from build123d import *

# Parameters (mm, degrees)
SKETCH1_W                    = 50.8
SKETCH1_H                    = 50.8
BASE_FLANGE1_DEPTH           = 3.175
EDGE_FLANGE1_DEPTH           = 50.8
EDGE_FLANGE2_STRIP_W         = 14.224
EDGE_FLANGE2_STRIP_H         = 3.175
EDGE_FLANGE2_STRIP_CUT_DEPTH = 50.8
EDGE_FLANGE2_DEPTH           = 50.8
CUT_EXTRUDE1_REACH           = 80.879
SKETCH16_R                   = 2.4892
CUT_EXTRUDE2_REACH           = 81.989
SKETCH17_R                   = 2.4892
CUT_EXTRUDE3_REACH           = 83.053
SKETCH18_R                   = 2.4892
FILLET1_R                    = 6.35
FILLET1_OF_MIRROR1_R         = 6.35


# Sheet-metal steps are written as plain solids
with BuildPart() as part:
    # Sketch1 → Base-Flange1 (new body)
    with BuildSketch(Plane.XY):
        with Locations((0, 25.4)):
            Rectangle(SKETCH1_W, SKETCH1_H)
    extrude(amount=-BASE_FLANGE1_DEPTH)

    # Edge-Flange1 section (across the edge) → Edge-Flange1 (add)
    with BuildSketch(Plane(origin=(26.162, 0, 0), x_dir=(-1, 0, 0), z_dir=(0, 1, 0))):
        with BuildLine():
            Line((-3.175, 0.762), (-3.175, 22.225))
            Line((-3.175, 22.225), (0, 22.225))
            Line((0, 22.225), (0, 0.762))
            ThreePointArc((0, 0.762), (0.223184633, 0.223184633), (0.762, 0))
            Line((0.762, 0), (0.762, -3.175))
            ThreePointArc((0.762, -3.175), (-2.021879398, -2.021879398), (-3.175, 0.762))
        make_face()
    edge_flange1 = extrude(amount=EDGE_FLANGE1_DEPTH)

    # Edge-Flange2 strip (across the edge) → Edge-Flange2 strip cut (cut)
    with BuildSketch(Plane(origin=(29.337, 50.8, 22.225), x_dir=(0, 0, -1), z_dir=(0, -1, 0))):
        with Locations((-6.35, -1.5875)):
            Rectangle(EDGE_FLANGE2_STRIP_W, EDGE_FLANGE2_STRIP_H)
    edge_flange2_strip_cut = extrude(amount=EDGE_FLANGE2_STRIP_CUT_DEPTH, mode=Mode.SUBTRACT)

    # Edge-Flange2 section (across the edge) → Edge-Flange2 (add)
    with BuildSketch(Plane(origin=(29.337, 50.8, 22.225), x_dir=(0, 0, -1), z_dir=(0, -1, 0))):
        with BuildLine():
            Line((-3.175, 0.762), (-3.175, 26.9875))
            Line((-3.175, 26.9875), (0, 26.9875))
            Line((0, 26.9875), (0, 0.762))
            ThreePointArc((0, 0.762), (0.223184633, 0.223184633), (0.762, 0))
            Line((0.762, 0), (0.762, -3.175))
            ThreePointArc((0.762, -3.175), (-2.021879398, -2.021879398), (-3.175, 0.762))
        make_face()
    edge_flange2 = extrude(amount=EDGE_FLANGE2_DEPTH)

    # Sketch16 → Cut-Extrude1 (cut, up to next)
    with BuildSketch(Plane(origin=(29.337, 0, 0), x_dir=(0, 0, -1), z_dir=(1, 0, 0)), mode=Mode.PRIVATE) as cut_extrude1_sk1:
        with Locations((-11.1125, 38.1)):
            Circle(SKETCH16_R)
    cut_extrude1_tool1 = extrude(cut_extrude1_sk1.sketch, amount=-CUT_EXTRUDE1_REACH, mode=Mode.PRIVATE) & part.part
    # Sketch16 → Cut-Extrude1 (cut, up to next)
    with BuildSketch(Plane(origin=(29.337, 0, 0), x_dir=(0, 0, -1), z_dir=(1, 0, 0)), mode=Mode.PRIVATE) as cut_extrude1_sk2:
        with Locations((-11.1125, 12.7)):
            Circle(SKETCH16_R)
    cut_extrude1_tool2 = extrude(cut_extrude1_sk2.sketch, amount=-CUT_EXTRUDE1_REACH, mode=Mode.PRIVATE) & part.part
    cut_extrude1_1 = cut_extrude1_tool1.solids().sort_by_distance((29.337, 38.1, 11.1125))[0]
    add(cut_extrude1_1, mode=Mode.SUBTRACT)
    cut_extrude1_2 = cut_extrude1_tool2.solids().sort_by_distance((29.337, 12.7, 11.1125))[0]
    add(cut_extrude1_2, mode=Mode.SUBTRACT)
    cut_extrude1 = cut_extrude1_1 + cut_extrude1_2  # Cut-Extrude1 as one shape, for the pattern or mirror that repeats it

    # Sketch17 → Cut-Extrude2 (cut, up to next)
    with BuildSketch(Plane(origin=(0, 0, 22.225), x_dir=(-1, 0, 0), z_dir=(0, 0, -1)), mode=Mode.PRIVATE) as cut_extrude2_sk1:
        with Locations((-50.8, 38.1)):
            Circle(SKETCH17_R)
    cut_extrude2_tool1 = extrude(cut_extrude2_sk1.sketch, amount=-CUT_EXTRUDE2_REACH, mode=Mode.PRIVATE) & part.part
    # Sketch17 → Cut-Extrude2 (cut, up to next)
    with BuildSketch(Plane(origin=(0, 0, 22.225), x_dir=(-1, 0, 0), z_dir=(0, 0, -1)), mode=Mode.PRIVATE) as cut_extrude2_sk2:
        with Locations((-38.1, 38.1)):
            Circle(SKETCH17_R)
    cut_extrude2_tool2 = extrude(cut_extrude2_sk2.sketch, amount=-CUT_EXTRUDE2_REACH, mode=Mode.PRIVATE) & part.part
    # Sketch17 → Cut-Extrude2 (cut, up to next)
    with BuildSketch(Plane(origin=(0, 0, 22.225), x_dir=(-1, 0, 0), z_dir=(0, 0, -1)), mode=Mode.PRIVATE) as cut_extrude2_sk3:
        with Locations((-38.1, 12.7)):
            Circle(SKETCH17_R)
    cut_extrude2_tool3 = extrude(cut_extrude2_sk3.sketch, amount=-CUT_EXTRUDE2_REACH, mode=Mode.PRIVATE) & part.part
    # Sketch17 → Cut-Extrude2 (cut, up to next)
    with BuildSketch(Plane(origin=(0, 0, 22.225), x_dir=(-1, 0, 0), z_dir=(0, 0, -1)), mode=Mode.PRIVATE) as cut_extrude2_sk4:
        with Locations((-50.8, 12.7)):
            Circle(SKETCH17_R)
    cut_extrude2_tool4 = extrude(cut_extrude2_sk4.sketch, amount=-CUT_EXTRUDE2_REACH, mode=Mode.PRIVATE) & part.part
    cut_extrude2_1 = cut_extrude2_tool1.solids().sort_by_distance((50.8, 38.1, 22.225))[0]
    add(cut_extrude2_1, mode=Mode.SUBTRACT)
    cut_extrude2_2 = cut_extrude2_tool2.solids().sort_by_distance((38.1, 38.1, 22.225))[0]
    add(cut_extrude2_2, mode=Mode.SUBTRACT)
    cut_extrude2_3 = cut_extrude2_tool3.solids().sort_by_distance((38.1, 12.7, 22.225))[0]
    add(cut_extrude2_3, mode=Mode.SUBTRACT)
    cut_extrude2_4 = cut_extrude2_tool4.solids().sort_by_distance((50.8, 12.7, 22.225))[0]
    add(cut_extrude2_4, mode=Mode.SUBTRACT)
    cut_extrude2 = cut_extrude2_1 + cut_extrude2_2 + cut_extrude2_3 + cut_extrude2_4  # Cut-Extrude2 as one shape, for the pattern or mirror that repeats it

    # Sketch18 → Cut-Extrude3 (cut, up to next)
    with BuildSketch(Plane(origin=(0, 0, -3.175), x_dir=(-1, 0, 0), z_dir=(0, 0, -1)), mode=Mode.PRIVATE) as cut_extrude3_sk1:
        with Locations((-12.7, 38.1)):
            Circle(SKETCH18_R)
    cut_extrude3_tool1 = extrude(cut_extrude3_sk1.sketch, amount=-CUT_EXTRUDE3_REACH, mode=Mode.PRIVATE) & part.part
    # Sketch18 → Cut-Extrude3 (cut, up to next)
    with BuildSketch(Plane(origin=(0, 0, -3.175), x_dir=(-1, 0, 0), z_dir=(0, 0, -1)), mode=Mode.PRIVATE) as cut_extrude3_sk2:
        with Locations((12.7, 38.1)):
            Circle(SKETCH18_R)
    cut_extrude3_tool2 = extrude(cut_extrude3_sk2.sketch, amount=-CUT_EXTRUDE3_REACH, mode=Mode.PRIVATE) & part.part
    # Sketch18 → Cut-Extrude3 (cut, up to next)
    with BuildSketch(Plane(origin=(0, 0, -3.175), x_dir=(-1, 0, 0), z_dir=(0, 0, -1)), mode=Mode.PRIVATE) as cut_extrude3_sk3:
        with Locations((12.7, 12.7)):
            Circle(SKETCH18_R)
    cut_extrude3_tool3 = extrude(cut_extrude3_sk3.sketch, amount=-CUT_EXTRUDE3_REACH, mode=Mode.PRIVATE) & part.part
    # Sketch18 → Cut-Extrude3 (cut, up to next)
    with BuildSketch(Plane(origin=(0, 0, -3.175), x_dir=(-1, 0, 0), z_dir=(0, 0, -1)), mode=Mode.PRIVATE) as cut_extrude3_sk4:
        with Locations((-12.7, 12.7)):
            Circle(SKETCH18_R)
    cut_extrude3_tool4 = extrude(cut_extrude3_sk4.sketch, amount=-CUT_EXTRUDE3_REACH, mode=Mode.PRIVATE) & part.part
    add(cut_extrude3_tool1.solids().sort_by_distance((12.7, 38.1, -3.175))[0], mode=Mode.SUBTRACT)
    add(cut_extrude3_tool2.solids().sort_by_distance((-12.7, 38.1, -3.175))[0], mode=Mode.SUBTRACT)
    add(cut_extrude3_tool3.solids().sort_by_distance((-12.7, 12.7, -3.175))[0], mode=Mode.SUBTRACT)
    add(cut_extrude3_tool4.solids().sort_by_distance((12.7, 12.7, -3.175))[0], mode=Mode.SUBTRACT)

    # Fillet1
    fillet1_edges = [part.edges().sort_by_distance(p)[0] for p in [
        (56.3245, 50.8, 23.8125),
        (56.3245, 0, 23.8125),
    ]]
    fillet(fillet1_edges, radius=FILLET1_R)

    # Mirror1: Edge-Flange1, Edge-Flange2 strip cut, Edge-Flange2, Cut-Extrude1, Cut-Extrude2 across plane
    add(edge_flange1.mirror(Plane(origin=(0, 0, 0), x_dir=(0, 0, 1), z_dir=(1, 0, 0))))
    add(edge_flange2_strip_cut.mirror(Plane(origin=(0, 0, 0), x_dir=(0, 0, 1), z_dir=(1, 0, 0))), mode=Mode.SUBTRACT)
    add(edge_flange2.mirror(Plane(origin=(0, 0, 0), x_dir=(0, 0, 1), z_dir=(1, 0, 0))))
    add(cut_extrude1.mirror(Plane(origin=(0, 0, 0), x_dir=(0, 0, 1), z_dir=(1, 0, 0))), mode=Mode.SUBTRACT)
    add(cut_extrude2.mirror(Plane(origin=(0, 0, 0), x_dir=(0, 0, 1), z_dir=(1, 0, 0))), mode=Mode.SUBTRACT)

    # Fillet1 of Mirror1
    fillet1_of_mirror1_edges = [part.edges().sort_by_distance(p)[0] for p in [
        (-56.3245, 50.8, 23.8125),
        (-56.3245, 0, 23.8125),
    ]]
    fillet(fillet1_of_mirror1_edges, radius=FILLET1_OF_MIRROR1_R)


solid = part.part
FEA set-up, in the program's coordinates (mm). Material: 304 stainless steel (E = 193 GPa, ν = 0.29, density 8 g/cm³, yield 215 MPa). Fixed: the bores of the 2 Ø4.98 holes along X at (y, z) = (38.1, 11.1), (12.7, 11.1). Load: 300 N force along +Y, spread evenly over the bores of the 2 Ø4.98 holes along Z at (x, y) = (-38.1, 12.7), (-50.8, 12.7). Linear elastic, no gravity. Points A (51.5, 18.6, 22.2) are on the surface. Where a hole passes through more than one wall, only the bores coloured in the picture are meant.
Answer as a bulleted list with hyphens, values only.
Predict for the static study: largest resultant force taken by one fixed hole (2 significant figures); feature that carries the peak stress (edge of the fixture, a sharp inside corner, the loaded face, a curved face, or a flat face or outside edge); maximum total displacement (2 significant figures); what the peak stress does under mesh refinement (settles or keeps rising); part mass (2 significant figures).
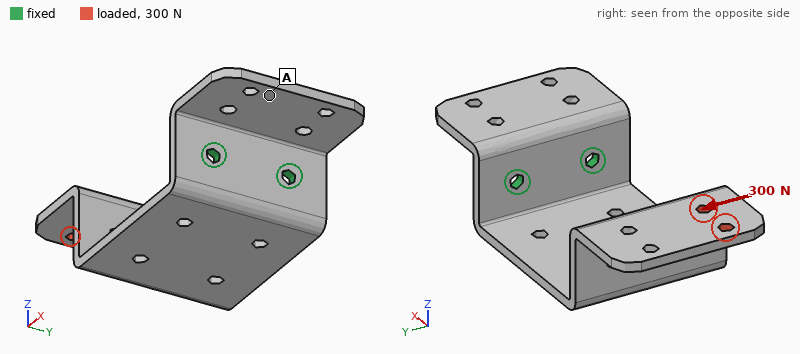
- 730 N
- edge of the fixture
- 0.50 mm
- keeps rising
- 200 g
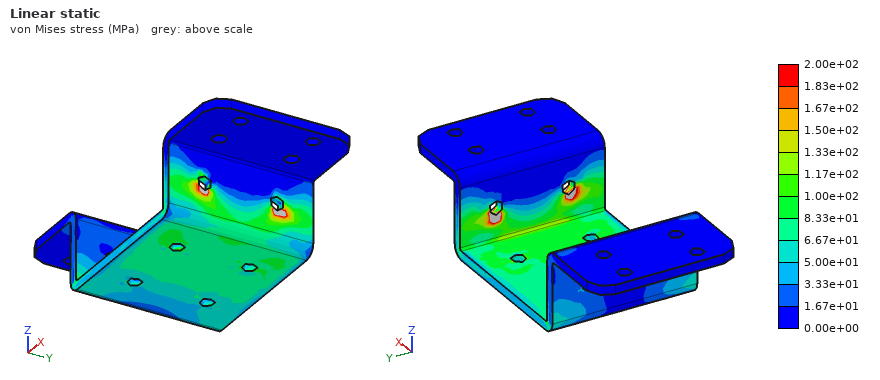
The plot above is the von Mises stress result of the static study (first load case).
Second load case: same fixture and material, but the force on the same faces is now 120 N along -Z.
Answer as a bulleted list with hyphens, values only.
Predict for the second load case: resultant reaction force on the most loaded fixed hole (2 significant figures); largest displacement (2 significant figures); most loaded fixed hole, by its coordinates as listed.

- 120 N
- 1.2 mm
- (12.7, 11.1)
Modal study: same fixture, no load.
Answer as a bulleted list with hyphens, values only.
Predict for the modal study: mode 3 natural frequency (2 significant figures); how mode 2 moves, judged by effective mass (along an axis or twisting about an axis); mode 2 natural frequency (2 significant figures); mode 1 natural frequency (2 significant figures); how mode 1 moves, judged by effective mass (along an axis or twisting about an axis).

- 970 Hz
- along Y
- 560 Hz
- 240 Hz
- along Z
